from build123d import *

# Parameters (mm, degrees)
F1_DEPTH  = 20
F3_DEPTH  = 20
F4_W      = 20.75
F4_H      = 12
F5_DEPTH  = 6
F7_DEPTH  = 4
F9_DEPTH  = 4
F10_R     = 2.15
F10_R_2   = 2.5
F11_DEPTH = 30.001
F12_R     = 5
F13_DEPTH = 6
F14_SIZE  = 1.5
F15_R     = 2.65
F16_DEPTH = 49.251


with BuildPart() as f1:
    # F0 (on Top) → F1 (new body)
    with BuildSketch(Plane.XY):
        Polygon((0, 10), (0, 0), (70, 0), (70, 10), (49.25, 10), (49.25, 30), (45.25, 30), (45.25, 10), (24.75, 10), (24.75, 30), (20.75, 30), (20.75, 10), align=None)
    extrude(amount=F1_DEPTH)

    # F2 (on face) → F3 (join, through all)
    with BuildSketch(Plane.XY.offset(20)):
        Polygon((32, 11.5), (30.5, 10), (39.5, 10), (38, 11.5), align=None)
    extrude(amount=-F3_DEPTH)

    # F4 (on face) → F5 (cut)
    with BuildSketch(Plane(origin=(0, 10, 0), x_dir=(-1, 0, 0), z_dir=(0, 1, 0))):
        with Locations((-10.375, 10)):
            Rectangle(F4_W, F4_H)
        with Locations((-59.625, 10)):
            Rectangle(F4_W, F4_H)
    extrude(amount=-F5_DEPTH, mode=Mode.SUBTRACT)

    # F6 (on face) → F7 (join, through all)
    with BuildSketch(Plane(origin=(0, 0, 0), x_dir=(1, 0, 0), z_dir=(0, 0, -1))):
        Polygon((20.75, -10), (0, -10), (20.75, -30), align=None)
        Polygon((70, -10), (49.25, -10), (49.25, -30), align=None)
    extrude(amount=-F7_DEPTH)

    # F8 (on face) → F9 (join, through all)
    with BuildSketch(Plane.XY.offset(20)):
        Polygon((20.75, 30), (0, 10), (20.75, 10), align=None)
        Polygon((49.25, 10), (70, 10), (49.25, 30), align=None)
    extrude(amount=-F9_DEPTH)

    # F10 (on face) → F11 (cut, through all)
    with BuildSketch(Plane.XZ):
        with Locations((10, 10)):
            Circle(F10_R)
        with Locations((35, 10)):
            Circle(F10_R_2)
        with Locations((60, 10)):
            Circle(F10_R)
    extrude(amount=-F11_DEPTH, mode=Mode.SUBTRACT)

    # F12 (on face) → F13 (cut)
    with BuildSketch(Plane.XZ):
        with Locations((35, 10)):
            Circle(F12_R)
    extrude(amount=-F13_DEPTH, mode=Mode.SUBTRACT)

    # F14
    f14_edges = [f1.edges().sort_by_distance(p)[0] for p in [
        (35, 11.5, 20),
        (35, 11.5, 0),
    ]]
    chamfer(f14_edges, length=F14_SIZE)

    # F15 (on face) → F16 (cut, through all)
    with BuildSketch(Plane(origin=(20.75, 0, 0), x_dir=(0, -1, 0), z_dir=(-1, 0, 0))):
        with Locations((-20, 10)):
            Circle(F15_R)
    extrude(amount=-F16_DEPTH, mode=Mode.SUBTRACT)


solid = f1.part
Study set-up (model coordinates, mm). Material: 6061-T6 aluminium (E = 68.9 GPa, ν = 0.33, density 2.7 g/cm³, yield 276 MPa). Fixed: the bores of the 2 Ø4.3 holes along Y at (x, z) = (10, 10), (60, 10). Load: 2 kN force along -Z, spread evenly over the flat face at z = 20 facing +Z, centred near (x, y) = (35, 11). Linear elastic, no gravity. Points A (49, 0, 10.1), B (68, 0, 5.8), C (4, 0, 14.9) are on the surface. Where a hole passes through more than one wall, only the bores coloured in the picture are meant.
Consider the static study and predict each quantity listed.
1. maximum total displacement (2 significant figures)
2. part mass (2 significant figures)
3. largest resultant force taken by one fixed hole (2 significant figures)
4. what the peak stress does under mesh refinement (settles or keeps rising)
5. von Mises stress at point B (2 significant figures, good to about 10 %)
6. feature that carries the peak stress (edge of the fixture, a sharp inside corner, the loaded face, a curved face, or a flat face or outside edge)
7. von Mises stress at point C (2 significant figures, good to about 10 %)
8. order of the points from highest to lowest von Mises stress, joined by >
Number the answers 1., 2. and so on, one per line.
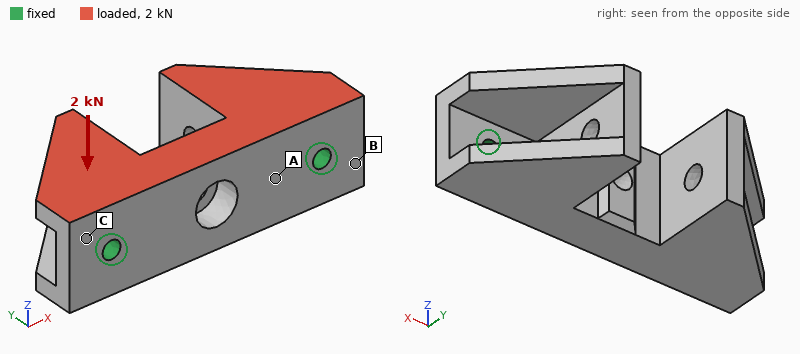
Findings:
1. 0.11 mm
2. 46 g
3. 1.0 kN
4. keeps rising
5. 32 MPa
6. edge of the fixture
7. 45 MPa
8. C > B > A
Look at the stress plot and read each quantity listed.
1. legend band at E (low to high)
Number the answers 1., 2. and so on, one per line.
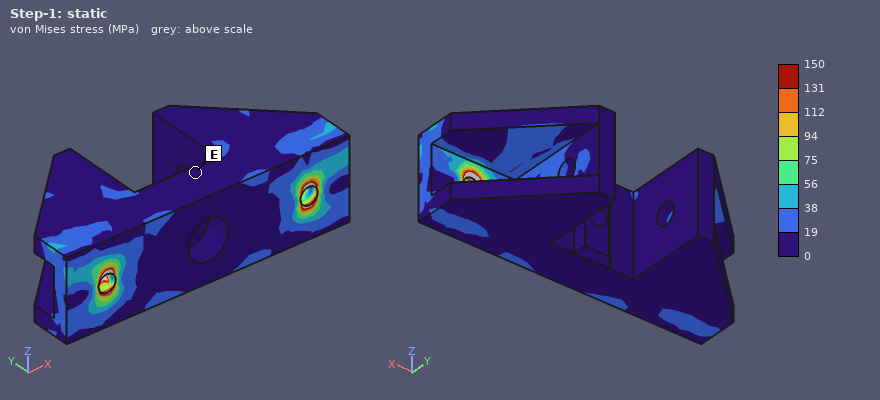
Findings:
1. 0 to 19 MPa
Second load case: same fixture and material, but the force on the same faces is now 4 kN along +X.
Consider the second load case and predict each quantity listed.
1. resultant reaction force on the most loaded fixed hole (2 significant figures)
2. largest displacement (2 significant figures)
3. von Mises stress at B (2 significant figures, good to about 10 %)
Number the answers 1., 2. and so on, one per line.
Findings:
1. 2.2 kN
2. 40 µm
3. 28 MPa
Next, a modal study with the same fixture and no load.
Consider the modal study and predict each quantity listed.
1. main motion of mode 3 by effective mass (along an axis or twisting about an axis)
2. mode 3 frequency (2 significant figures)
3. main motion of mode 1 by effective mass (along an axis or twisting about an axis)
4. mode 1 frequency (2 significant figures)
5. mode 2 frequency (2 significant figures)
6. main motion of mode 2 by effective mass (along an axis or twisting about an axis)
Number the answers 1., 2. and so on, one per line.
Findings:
1. twisting about Y
2. 8900 Hz
3. along Z
4. 4100 Hz
5. 7500 Hz
6. along Y
